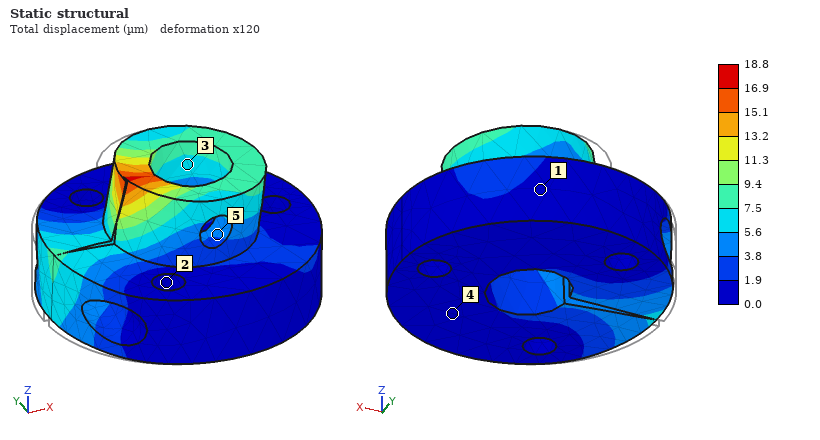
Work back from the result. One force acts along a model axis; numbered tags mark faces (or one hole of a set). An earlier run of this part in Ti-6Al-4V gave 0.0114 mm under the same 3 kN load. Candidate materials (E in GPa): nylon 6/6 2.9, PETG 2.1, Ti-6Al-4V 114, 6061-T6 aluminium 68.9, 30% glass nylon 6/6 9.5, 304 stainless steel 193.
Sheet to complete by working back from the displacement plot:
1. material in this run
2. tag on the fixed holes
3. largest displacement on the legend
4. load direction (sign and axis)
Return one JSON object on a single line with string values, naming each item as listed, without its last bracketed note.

{"material in this run": "6061-T6 aluminium", "tag on the fixed holes": "2", "largest displacement on the legend": "18.8 µm", "load direction": "+X"}
